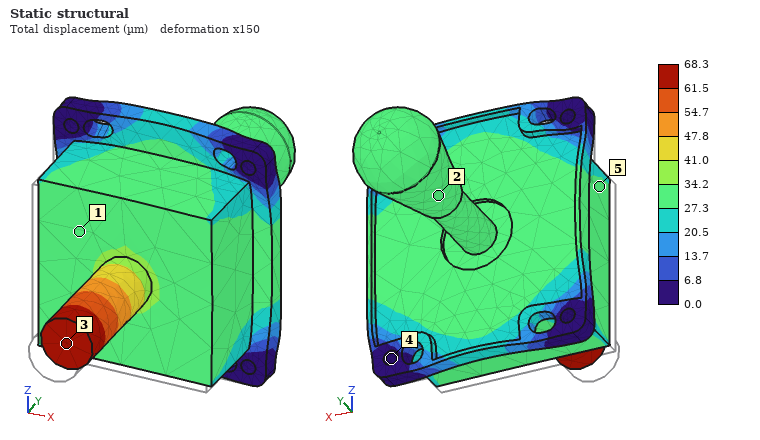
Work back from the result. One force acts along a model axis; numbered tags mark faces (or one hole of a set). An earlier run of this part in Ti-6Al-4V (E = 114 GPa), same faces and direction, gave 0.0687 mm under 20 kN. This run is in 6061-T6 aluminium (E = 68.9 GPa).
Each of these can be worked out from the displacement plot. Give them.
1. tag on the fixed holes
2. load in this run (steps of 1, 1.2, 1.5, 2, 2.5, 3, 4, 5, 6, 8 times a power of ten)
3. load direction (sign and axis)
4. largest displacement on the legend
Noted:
4
12 kN
+Y
68.3 µm
